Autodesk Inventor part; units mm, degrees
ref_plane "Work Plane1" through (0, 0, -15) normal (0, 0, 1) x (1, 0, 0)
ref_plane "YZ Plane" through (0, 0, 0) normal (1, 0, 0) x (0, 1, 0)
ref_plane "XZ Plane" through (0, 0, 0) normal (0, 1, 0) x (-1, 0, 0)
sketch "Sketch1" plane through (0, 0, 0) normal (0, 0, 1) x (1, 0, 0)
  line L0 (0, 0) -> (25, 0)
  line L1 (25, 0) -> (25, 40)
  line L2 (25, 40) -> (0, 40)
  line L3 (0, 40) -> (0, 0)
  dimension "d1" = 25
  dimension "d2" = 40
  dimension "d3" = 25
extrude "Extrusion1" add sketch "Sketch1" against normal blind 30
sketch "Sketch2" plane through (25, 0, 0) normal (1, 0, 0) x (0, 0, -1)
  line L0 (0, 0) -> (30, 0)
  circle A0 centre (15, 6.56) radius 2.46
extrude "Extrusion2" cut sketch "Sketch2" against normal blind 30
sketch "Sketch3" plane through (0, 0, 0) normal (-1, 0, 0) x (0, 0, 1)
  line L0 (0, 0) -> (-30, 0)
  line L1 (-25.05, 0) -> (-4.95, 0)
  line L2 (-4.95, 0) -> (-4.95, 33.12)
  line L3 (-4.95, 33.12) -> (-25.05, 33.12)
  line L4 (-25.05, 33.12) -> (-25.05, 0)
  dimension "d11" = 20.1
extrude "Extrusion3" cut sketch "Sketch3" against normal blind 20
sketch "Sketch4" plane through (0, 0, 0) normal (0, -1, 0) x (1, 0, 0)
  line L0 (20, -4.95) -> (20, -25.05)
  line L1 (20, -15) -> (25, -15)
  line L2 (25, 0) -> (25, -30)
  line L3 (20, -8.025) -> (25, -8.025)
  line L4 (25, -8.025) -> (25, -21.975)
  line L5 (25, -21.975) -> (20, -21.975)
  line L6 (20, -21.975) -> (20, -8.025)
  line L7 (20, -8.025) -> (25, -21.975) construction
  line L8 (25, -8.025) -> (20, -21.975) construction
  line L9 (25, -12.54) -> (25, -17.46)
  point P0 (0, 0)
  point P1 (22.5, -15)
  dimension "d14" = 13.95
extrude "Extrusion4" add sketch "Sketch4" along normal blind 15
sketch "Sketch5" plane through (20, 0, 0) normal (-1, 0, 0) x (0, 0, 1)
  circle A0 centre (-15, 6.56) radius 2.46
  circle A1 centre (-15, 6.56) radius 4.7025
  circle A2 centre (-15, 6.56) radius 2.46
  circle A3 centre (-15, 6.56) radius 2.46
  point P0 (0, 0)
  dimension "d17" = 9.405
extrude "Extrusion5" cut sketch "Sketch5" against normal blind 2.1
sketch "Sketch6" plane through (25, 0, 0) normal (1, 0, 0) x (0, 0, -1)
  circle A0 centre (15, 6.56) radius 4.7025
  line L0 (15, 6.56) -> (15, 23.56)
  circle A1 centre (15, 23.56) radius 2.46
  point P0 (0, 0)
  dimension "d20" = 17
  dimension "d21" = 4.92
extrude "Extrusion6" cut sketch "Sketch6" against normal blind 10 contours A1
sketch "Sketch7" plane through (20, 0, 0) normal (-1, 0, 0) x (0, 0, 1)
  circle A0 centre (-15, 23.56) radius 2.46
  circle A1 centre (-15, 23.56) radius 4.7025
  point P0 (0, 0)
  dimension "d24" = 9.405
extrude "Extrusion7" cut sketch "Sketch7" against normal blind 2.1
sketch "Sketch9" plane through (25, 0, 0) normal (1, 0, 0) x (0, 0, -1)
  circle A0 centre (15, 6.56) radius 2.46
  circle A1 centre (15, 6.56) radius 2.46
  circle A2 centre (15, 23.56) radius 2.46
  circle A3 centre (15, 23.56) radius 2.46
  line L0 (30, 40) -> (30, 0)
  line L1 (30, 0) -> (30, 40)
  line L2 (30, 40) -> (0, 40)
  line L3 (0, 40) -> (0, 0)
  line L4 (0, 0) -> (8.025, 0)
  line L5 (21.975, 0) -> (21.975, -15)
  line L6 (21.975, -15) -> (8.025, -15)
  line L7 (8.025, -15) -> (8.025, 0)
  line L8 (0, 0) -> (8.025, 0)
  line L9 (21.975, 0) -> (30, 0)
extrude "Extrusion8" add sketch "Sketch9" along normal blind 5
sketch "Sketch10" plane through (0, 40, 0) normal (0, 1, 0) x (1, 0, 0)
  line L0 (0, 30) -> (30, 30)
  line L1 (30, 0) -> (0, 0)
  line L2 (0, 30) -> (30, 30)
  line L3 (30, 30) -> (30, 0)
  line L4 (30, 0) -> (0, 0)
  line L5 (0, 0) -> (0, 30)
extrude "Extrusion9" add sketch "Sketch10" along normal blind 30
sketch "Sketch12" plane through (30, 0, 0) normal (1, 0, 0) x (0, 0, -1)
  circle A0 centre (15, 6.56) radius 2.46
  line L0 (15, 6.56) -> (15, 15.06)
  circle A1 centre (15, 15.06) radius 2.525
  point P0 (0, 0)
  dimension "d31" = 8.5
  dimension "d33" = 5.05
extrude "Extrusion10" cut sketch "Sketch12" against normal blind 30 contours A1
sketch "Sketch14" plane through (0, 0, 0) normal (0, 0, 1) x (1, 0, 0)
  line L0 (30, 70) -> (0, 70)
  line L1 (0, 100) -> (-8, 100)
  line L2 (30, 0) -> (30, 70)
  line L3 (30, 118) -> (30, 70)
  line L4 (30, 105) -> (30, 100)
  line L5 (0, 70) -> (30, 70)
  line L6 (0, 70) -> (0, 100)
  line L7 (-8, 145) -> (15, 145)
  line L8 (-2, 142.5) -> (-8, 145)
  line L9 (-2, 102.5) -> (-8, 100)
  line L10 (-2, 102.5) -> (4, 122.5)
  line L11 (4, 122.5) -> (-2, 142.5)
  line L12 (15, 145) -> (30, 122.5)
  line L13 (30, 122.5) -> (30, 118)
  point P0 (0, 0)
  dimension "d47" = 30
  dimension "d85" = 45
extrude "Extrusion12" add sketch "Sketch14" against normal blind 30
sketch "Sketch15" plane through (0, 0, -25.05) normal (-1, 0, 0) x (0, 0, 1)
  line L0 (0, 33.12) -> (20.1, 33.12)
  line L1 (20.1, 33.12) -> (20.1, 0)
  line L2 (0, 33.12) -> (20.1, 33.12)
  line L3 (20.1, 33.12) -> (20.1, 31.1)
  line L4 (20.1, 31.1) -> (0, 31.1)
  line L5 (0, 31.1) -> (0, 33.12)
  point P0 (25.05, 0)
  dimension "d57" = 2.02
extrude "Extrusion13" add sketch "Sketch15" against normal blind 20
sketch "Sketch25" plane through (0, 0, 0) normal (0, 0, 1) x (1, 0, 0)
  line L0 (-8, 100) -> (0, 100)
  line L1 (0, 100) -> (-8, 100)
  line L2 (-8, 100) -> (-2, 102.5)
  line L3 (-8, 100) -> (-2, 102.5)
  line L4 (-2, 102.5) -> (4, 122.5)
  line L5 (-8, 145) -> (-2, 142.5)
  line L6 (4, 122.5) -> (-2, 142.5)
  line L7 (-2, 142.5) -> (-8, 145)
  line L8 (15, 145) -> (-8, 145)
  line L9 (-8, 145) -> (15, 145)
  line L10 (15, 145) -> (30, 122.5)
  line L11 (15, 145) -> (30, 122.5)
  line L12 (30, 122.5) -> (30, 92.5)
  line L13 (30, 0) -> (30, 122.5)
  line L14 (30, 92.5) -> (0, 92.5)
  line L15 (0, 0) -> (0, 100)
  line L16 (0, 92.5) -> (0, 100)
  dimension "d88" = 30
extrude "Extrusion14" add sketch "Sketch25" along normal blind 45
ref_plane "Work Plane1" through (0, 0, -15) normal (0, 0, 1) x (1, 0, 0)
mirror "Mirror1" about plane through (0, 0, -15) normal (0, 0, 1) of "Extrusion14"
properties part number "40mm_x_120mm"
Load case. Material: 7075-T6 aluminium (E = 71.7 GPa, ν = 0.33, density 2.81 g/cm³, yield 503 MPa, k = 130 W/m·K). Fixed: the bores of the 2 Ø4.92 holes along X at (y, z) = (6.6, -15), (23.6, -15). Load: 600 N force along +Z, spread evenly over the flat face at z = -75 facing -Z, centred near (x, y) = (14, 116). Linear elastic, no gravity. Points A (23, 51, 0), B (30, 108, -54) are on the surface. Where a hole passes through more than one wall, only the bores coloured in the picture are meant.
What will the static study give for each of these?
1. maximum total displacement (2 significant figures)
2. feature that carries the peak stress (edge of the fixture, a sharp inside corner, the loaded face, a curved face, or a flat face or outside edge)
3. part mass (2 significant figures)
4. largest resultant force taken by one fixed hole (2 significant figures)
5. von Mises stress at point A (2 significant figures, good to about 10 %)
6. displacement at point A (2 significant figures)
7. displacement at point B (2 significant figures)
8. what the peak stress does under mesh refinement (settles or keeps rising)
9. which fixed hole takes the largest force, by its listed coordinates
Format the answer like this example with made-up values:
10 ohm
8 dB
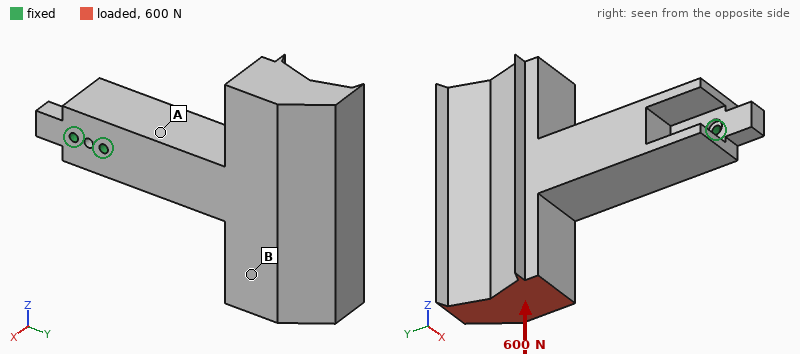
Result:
0.16 mm
edge of the fixture
670 g
3.0 kN
10.0 MPa
0.029 mm
0.10 mm
keeps rising
(23.6, -15)
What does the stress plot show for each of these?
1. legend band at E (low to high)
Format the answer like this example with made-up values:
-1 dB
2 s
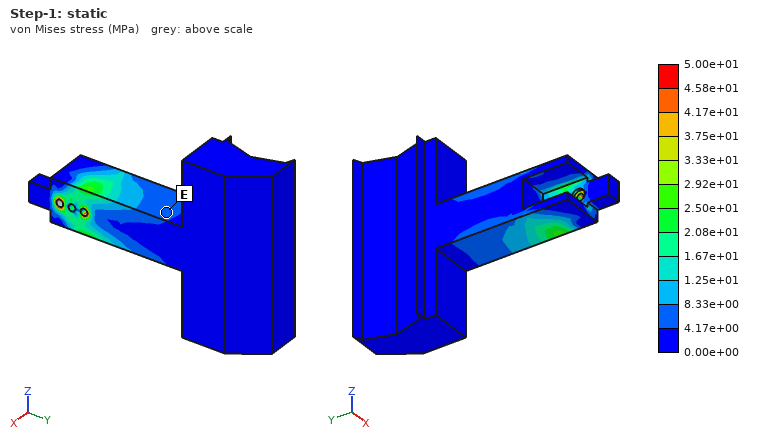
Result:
4.17e+00 to 8.33e+00 MPa
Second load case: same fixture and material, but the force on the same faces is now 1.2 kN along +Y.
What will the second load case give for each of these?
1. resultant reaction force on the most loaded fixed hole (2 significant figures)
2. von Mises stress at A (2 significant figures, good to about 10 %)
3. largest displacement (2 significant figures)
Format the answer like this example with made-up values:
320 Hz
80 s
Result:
3.3 kN
17 MPa
0.27 mm
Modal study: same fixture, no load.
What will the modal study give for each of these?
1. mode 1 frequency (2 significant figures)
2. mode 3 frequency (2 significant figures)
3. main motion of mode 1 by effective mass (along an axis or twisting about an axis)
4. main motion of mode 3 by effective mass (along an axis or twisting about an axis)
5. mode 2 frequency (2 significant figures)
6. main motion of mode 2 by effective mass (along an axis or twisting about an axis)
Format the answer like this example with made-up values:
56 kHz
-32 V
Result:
460 Hz
780 Hz
along X
twisting about Y
500 Hz
along Z
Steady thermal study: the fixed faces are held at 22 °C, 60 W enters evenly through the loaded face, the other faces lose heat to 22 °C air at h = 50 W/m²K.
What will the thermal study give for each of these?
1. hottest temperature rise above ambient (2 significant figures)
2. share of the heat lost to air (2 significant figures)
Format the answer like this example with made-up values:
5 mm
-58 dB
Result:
40 K
60 %
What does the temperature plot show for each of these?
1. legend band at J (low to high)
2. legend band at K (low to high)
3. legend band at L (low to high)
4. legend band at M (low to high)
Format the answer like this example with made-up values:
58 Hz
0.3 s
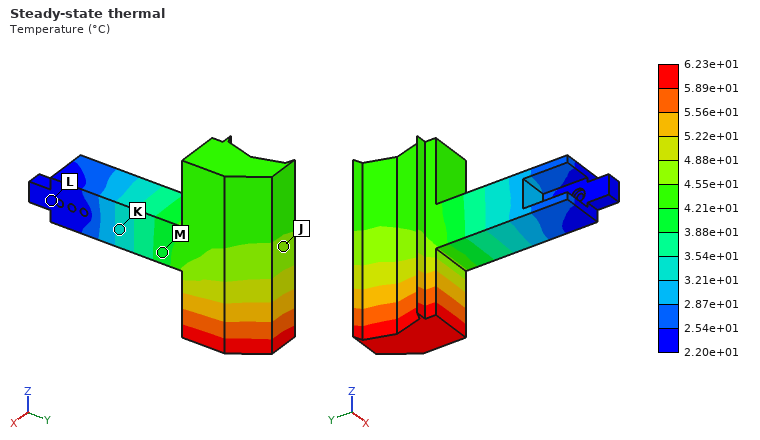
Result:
4.55e+01 to 4.88e+01 °C
3.21e+01 to 3.54e+01 °C
2.20e+01 to 2.54e+01 °C
3.88e+01 to 4.21e+01 °C
